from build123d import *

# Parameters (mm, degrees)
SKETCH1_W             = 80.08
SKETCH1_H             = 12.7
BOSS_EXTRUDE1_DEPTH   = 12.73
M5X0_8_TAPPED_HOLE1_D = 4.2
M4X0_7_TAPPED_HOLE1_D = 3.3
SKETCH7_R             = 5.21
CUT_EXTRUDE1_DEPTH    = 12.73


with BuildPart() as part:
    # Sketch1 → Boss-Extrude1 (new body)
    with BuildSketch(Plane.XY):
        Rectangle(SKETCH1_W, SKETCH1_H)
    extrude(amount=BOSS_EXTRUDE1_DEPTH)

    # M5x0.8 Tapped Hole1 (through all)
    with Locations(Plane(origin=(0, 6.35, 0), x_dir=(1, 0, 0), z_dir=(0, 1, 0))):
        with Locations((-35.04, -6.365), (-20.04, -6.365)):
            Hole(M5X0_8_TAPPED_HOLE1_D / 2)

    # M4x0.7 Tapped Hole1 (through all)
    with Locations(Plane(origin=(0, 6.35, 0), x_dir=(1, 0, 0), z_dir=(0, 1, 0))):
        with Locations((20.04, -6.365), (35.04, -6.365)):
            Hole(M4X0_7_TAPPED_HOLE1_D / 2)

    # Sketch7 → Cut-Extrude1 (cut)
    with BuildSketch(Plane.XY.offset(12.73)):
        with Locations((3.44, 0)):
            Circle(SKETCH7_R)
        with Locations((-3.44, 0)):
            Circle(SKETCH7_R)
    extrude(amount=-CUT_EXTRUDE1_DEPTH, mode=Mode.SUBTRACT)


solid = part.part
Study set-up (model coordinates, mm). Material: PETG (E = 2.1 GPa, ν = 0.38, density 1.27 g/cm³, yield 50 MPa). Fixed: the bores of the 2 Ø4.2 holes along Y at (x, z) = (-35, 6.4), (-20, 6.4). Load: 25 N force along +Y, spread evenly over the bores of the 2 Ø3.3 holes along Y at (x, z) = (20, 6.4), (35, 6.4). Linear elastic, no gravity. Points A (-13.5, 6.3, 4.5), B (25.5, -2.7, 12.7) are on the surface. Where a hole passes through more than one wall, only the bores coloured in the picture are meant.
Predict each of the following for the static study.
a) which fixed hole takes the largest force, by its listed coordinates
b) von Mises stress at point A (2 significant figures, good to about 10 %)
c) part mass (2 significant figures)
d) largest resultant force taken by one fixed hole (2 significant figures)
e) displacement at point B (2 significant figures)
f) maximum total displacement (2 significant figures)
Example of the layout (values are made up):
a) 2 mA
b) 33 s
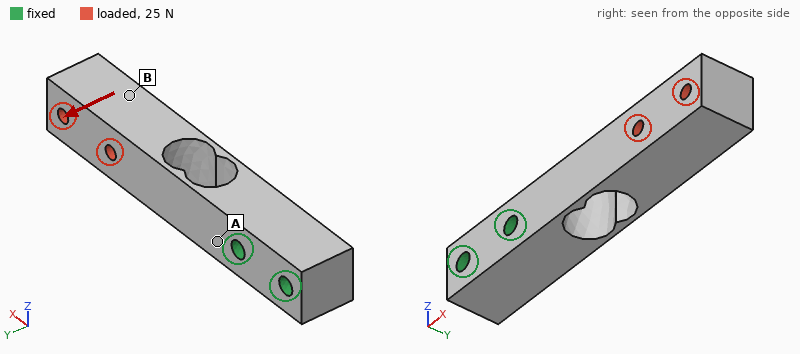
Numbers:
a) (-20, 6.4)
b) 3.8 MPa
c) 13 g
d) 35 N
e) 0.70 mm
f) 0.84 mm
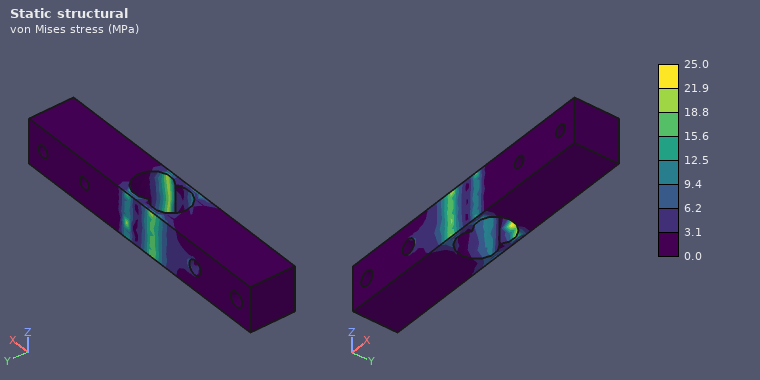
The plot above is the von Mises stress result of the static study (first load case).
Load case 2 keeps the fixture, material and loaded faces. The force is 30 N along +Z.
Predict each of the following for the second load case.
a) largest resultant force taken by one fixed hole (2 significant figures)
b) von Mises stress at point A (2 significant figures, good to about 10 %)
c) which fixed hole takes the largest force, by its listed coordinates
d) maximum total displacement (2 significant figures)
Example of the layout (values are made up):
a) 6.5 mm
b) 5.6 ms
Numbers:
a) 74 N
b) 1.7 MPa
c) (-20, 6.4)
d) 0.97 mm
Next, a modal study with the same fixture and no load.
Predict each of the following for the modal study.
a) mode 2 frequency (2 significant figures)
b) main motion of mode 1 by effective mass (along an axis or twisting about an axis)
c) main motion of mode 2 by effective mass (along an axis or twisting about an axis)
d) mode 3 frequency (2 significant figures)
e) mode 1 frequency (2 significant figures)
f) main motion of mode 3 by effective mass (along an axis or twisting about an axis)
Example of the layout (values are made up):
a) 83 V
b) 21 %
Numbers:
a) 440 Hz
b) along Y
c) along Z
d) 1700 Hz
e) 380 Hz
f) twisting about X
